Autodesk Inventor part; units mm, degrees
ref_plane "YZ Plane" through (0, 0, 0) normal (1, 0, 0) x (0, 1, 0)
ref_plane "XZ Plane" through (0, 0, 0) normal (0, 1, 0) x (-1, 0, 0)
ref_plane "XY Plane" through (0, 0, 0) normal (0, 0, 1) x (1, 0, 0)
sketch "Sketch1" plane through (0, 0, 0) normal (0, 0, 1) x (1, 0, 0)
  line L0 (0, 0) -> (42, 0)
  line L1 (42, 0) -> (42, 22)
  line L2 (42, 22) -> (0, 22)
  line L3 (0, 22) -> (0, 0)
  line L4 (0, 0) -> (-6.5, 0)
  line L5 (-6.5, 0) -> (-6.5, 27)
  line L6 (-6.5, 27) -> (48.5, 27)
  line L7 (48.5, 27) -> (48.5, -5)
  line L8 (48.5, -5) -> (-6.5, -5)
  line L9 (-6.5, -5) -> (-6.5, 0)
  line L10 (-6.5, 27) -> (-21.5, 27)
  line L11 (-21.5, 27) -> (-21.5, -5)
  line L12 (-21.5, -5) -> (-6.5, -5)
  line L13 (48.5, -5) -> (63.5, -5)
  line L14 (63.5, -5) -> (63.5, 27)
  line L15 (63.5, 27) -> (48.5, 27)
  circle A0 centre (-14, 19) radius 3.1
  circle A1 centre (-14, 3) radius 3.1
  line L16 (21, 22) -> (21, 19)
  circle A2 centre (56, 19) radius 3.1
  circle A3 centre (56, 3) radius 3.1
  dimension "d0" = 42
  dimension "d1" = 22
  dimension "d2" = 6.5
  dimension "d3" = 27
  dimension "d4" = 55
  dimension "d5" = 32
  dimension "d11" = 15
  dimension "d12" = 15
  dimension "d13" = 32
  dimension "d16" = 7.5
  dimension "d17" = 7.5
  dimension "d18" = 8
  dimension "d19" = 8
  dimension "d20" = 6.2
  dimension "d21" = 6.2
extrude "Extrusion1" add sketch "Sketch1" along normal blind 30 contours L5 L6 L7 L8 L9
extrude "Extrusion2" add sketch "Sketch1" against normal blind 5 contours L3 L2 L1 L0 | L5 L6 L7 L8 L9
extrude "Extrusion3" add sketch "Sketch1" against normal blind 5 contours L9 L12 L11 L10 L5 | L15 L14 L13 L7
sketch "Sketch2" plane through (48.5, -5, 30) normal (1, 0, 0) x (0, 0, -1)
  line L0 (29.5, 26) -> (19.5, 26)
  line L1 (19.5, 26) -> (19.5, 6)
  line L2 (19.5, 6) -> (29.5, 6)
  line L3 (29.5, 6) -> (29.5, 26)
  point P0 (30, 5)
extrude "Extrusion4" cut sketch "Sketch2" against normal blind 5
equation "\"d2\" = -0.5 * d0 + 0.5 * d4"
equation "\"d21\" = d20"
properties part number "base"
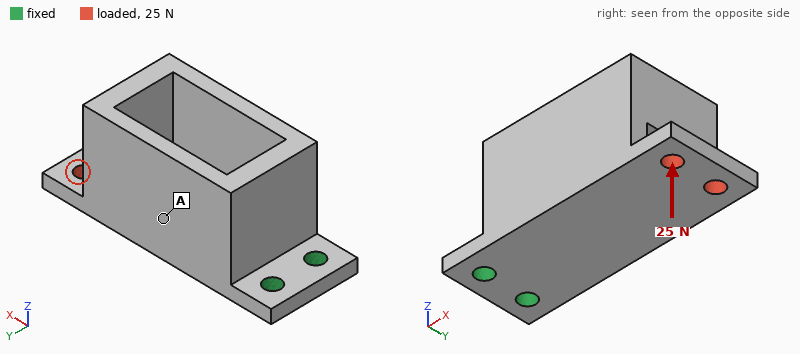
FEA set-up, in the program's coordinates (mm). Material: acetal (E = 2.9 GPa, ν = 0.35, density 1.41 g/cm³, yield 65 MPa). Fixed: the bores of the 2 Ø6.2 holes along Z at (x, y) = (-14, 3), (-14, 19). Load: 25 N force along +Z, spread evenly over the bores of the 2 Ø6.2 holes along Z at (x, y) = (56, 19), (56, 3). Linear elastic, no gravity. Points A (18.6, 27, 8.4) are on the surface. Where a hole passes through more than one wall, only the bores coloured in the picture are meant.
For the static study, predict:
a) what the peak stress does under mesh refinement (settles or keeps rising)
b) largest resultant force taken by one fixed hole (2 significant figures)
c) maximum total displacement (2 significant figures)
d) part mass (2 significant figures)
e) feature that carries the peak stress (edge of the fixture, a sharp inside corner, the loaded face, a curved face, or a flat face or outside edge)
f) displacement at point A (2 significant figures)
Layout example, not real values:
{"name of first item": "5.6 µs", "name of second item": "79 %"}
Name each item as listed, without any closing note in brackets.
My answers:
{"what the peak stress does under mesh refinement": "keeps rising", "largest resultant force taken by one fixed hole": "13 N", "maximum total displacement": "1.0 mm", "part mass": "52 g", "feature that carries the peak stress": "edge of the fixture", "displacement at point A": "0.40 mm"}
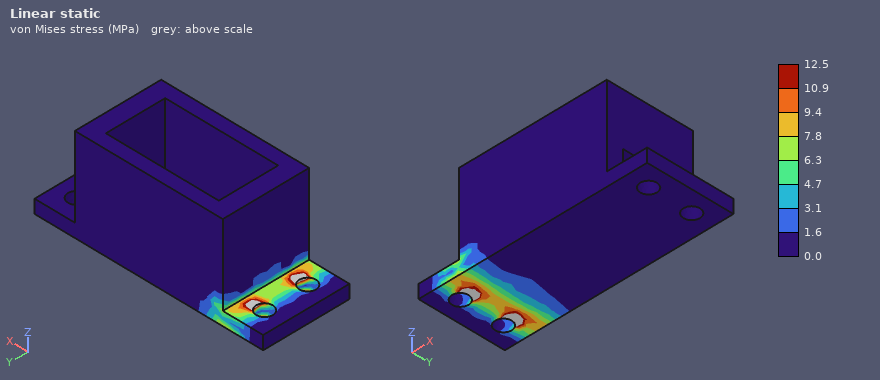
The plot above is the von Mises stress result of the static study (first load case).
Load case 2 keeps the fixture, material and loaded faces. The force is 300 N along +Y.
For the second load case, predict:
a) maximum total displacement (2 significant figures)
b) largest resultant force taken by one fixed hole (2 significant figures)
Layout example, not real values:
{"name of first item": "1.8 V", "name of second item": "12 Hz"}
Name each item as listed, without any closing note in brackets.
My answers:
{"maximum total displacement": "0.96 mm", "largest resultant force taken by one fixed hole": "1.0 kN"}
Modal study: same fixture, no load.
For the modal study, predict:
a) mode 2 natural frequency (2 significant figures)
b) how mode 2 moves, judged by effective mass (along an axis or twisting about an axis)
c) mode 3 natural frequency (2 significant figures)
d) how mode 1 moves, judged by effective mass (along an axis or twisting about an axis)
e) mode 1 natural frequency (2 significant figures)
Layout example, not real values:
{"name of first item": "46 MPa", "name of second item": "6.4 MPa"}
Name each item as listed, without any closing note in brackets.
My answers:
{"mode 2 natural frequency": "660 Hz", "how mode 2 moves, judged by effective mass": "along Y", "mode 3 natural frequency": "1000 Hz", "how mode 1 moves, judged by effective mass": "along Z", "mode 1 natural frequency": "190 Hz"}
